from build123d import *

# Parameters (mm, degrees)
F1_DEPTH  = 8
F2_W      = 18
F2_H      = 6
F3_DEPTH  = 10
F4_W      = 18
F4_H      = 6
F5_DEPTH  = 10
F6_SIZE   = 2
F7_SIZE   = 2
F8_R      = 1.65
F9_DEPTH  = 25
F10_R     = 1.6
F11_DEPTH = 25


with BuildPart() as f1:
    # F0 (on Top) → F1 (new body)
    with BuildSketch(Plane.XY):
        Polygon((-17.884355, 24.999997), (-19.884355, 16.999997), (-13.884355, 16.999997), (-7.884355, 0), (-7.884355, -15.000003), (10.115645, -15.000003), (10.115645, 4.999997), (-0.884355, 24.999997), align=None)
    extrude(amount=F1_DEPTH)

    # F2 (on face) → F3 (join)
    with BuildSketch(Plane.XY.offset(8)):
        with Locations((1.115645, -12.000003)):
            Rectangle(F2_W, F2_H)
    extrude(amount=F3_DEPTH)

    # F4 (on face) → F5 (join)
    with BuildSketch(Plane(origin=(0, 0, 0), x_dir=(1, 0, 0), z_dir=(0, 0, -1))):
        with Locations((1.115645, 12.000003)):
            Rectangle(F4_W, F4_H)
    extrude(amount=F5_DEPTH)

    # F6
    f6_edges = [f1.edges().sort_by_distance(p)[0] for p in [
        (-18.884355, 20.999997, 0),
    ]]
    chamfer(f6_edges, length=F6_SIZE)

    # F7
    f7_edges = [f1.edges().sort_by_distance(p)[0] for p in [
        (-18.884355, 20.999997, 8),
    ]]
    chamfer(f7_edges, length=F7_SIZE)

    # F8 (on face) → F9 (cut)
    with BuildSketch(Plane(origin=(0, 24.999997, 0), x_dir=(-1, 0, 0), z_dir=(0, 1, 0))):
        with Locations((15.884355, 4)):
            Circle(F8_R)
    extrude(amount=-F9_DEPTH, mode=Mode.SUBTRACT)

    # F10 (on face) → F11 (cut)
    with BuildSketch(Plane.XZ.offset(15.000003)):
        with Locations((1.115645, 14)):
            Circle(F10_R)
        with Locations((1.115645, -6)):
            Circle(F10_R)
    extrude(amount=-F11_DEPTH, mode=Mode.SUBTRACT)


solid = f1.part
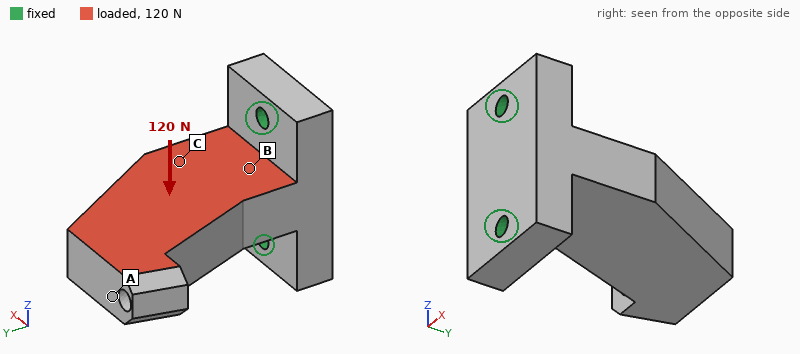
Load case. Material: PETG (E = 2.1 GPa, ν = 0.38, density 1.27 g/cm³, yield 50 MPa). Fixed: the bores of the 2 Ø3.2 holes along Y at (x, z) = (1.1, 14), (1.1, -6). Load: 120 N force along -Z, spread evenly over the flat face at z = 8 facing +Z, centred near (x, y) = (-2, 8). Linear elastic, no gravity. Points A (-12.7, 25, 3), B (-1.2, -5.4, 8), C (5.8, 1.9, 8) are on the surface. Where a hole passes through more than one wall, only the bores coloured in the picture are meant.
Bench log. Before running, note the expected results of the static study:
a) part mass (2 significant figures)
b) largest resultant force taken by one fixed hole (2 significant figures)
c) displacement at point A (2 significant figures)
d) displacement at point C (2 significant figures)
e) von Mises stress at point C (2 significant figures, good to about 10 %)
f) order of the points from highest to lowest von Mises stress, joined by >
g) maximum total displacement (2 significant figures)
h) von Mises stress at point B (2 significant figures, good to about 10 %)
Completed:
10 g
150 N
0.63 mm
0.14 mm
4.9 MPa
B > C > A
0.66 mm
8.7 MPa
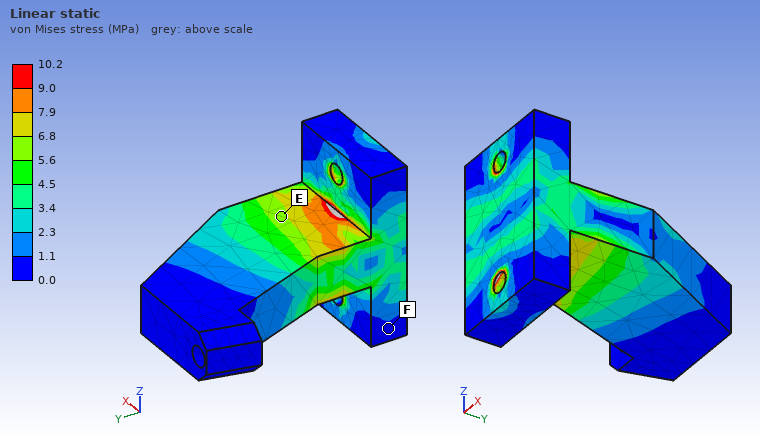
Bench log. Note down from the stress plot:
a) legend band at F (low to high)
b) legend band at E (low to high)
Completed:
0.0 to 1.1 MPa
5.6 to 6.8 MPa
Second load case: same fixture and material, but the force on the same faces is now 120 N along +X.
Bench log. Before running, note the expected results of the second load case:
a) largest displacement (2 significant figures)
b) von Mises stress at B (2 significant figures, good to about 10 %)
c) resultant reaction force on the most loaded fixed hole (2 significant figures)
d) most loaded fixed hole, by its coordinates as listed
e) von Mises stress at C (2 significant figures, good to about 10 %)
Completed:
0.59 mm
4.0 MPa
83 N
(1.1, 14)
3.0 MPa
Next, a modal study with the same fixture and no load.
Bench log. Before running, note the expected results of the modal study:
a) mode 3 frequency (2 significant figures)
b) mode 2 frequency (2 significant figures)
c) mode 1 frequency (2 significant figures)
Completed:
3500 Hz
1100 Hz
1100 Hz
